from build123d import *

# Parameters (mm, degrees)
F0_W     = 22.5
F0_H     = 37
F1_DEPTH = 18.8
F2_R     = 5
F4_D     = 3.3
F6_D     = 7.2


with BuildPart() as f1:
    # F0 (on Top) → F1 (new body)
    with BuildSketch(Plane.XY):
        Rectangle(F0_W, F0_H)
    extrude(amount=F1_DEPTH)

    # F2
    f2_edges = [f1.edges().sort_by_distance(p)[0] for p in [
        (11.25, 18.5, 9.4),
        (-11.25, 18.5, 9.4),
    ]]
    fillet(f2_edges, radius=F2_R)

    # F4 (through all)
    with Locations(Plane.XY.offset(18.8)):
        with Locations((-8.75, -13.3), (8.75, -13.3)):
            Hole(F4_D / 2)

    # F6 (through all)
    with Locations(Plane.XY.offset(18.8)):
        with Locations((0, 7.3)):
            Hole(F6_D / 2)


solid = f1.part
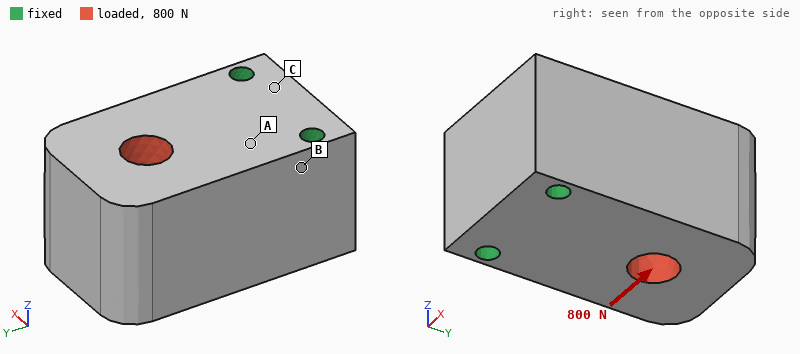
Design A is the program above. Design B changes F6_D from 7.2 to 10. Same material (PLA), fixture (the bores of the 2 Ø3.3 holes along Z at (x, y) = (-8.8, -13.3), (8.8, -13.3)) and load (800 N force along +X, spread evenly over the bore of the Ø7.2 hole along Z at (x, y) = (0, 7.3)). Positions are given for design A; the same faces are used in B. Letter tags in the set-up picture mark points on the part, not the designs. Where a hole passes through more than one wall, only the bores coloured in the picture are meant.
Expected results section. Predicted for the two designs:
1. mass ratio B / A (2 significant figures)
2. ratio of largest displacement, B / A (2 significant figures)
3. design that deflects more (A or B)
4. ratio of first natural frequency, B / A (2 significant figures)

0.95
1.2
B
1.0
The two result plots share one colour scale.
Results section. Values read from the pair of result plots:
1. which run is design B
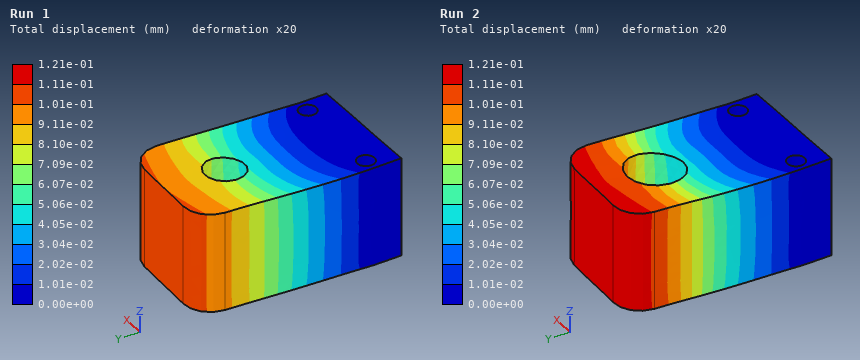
Run 2
